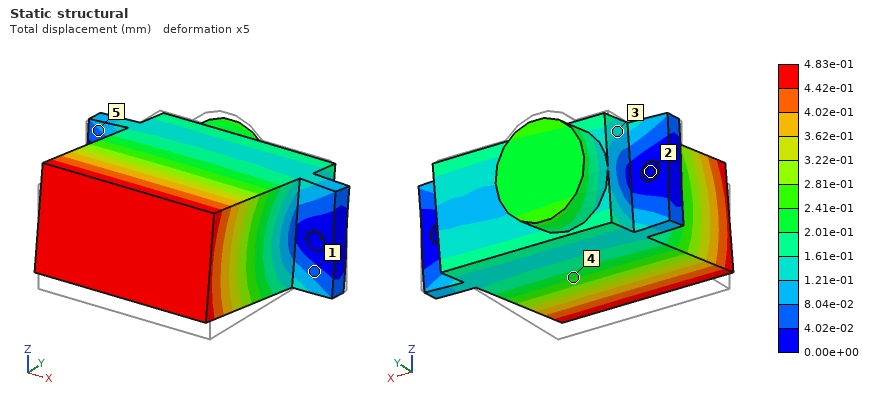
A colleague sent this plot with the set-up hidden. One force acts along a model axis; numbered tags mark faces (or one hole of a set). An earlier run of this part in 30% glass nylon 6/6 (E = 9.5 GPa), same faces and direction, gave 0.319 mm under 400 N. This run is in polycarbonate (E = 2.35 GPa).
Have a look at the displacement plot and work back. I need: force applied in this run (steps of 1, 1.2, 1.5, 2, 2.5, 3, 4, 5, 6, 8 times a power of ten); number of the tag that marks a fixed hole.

150 N
2
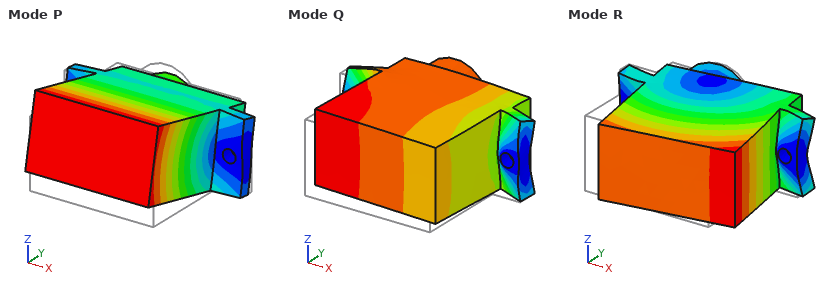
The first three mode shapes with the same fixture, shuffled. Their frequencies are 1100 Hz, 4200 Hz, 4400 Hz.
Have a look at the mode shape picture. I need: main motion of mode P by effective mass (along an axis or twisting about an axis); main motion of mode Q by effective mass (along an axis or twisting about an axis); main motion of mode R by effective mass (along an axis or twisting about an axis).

along Z
along Y
along X
